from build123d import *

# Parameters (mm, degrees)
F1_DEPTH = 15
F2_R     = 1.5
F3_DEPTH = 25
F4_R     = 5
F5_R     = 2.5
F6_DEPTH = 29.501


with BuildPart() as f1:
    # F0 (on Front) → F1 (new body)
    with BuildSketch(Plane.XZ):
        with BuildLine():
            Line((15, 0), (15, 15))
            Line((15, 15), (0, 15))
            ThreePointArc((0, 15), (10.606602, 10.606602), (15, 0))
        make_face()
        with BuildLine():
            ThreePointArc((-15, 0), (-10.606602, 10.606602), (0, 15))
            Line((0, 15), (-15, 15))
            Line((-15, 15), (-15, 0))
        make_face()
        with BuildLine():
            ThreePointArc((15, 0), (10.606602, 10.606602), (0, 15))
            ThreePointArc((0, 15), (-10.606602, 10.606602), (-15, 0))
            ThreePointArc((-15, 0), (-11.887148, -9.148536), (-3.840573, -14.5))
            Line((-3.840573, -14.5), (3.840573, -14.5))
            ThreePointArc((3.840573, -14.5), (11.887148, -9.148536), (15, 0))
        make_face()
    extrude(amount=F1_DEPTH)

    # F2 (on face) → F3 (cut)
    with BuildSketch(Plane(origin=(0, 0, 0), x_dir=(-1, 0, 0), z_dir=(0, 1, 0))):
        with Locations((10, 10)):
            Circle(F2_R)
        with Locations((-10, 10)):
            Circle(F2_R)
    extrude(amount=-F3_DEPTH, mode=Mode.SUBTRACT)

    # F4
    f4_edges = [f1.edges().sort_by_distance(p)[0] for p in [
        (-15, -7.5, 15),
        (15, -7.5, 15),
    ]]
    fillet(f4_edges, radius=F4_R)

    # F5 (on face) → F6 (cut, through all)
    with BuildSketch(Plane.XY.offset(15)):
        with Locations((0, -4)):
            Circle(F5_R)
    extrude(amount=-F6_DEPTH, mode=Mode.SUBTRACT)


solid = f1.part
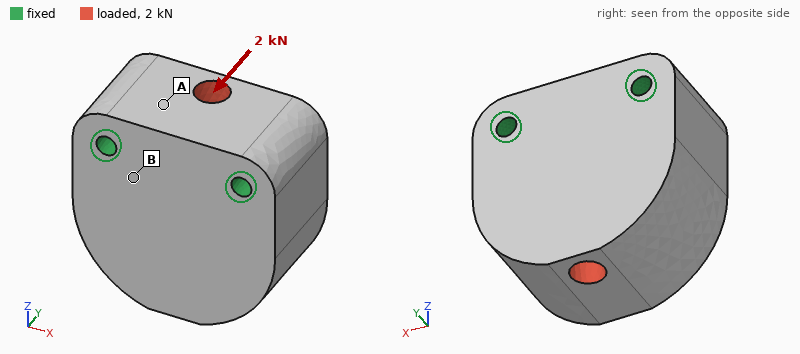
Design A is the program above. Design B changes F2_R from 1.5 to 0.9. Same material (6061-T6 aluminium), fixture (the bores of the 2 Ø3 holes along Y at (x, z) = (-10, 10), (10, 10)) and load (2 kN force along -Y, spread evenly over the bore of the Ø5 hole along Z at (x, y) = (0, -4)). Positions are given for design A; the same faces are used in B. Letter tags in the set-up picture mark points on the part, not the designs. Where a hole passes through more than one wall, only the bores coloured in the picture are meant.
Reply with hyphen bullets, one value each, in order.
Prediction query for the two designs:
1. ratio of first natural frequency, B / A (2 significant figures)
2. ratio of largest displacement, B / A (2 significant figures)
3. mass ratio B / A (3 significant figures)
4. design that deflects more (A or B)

- 0.90
- 1.2
- 1.01
- B
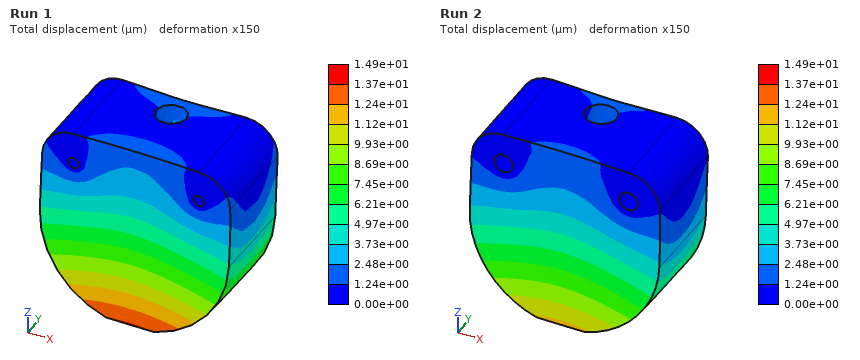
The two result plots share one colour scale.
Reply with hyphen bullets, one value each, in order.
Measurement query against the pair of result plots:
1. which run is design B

- Run 1
